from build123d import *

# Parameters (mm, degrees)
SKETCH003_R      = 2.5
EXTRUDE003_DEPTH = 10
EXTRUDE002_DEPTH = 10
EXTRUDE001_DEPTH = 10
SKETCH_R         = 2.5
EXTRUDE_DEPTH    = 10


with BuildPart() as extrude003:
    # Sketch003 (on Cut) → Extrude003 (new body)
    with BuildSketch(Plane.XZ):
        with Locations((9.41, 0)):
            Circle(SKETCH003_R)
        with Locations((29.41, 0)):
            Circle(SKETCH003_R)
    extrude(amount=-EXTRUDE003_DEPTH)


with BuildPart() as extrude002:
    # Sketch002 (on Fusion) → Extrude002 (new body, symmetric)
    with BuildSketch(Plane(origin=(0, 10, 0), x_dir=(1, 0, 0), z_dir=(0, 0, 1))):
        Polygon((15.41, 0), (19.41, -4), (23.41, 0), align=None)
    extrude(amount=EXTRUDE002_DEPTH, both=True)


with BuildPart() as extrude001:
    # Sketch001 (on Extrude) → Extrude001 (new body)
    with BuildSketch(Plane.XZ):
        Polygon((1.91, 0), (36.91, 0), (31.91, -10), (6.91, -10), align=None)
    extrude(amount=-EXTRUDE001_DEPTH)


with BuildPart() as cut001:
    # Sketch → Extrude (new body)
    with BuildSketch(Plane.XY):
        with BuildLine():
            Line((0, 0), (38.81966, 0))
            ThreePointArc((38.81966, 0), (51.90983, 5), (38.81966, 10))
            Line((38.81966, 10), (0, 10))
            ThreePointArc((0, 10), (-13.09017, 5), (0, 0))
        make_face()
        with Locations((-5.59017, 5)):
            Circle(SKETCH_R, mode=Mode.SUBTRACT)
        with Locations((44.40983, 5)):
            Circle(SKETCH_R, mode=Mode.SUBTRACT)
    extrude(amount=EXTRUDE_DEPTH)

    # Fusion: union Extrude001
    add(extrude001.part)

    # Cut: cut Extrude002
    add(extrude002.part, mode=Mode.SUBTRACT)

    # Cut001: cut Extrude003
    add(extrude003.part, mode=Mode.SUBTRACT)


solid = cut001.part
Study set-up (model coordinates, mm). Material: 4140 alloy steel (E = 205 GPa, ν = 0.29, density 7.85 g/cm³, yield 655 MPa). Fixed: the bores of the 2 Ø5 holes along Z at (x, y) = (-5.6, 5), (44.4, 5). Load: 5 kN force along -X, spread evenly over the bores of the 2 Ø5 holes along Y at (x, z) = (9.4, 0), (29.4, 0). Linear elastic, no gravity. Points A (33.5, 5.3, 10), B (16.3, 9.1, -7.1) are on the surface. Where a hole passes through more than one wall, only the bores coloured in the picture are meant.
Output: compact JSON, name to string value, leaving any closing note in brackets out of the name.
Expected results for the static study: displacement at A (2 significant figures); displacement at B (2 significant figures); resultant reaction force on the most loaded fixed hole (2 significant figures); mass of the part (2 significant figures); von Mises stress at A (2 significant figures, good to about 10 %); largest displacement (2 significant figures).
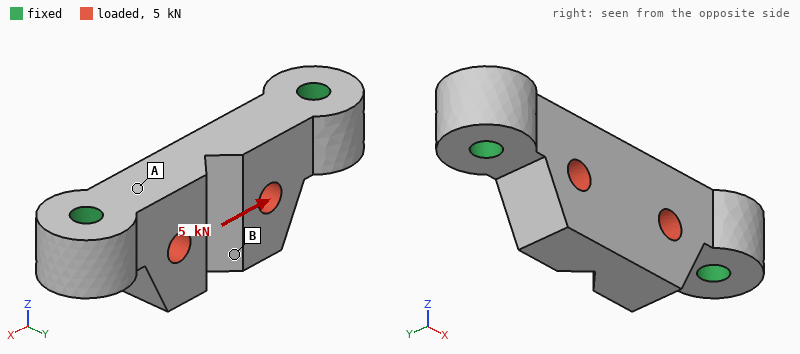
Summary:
{"displacement at A": "0.97 µm", "displacement at B": "2.6 µm", "resultant reaction force on the most loaded fixed hole": "2.6 kN", "mass of the part": "71 g", "von Mises stress at A": "12 MPa", "largest displacement": "2.9 µm"}
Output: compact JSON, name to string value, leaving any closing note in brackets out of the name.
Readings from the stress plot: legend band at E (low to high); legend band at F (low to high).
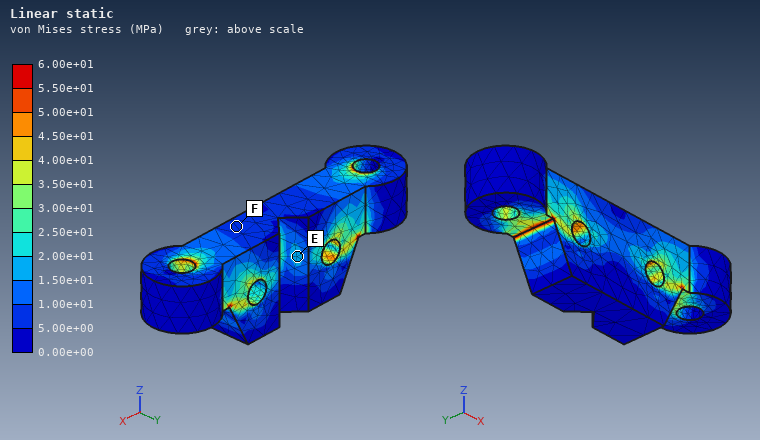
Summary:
{"legend band at E": "1.50e+01 to 2.00e+01 MPa", "legend band at F": "5.00e+00 to 1.00e+01 MPa"}
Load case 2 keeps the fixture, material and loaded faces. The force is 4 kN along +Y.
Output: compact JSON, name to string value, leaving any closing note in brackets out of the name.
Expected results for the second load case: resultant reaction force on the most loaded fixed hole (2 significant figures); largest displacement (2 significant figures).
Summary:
{"resultant reaction force on the most loaded fixed hole": "2.0 kN", "largest displacement": "24 µm"}
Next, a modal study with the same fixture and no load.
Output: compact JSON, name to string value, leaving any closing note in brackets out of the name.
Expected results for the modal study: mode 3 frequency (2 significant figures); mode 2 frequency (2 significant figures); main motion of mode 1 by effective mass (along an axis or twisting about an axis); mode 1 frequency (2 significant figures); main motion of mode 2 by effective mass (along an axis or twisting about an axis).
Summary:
{"mode 3 frequency": "21 kHz", "mode 2 frequency": "19 kHz", "main motion of mode 1 by effective mass": "along Y", "mode 1 frequency": "11 kHz", "main motion of mode 2 by effective mass": "along Z"}
